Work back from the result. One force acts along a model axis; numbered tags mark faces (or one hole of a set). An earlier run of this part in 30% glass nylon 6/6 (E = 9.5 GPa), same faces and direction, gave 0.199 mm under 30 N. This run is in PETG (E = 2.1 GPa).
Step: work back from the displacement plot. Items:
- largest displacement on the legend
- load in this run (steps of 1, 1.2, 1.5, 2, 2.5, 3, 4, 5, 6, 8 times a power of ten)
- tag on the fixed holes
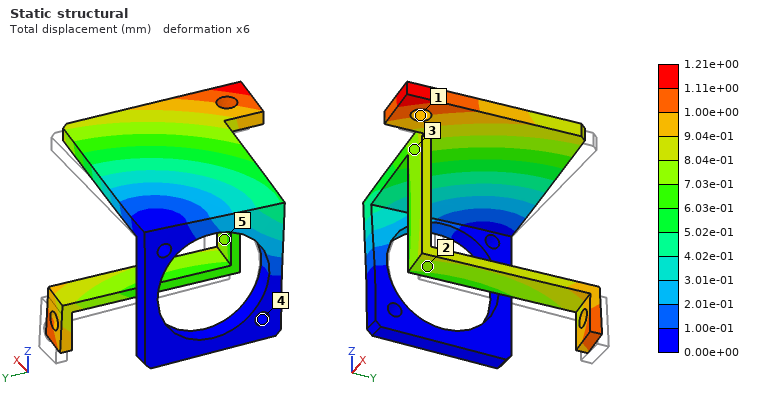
1.21e+00 mm
40 N
4
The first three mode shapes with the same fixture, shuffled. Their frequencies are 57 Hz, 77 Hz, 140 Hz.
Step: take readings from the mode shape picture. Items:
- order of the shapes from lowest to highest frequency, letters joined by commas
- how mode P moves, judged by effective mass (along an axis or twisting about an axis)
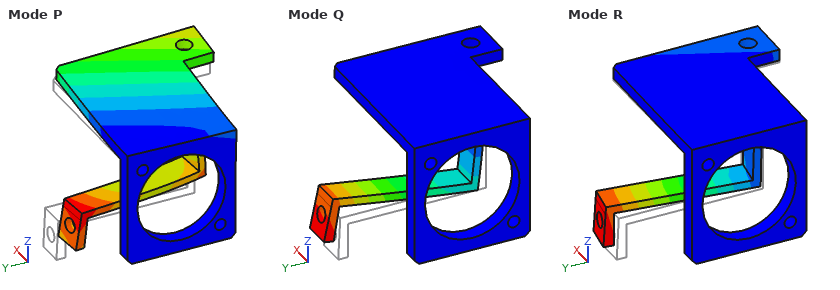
Q, R, P
along Z
